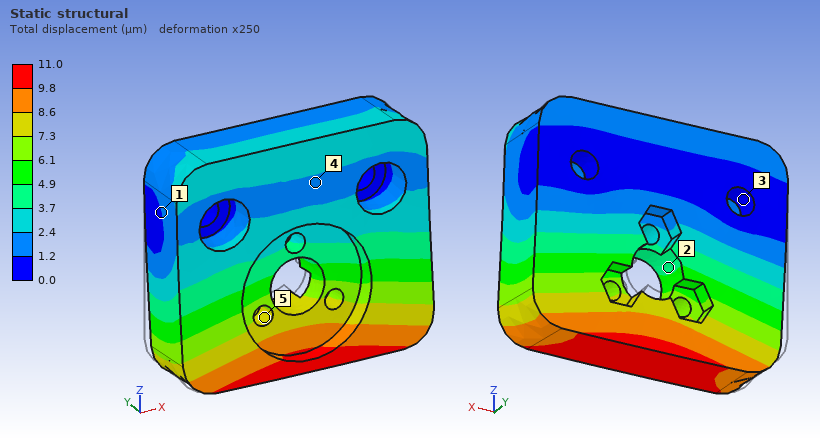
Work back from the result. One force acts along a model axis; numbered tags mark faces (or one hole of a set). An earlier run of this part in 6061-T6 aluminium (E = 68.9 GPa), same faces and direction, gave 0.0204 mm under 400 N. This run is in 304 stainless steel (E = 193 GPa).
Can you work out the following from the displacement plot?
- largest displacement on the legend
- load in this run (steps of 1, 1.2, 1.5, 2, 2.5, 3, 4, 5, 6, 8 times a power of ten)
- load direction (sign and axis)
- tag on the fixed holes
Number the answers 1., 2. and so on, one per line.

1. 11.0 µm
2. 600 N
3. -Y
4. 3
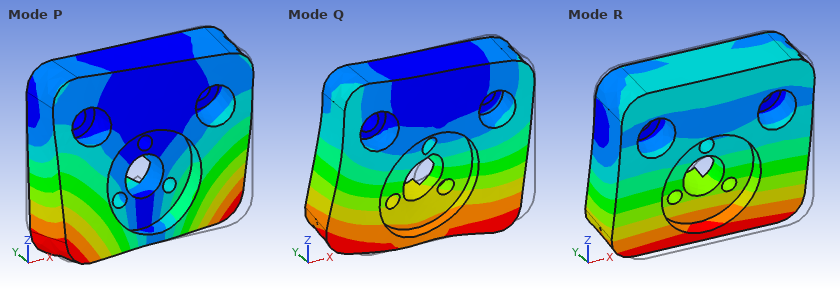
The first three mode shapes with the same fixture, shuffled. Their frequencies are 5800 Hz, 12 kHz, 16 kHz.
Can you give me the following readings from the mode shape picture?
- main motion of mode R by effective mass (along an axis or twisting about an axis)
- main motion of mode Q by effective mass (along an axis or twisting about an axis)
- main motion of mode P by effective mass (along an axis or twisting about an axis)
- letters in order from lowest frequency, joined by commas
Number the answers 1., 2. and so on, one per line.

1. along Y
2. along X
3. twisting about Z
4. R, P, Q
